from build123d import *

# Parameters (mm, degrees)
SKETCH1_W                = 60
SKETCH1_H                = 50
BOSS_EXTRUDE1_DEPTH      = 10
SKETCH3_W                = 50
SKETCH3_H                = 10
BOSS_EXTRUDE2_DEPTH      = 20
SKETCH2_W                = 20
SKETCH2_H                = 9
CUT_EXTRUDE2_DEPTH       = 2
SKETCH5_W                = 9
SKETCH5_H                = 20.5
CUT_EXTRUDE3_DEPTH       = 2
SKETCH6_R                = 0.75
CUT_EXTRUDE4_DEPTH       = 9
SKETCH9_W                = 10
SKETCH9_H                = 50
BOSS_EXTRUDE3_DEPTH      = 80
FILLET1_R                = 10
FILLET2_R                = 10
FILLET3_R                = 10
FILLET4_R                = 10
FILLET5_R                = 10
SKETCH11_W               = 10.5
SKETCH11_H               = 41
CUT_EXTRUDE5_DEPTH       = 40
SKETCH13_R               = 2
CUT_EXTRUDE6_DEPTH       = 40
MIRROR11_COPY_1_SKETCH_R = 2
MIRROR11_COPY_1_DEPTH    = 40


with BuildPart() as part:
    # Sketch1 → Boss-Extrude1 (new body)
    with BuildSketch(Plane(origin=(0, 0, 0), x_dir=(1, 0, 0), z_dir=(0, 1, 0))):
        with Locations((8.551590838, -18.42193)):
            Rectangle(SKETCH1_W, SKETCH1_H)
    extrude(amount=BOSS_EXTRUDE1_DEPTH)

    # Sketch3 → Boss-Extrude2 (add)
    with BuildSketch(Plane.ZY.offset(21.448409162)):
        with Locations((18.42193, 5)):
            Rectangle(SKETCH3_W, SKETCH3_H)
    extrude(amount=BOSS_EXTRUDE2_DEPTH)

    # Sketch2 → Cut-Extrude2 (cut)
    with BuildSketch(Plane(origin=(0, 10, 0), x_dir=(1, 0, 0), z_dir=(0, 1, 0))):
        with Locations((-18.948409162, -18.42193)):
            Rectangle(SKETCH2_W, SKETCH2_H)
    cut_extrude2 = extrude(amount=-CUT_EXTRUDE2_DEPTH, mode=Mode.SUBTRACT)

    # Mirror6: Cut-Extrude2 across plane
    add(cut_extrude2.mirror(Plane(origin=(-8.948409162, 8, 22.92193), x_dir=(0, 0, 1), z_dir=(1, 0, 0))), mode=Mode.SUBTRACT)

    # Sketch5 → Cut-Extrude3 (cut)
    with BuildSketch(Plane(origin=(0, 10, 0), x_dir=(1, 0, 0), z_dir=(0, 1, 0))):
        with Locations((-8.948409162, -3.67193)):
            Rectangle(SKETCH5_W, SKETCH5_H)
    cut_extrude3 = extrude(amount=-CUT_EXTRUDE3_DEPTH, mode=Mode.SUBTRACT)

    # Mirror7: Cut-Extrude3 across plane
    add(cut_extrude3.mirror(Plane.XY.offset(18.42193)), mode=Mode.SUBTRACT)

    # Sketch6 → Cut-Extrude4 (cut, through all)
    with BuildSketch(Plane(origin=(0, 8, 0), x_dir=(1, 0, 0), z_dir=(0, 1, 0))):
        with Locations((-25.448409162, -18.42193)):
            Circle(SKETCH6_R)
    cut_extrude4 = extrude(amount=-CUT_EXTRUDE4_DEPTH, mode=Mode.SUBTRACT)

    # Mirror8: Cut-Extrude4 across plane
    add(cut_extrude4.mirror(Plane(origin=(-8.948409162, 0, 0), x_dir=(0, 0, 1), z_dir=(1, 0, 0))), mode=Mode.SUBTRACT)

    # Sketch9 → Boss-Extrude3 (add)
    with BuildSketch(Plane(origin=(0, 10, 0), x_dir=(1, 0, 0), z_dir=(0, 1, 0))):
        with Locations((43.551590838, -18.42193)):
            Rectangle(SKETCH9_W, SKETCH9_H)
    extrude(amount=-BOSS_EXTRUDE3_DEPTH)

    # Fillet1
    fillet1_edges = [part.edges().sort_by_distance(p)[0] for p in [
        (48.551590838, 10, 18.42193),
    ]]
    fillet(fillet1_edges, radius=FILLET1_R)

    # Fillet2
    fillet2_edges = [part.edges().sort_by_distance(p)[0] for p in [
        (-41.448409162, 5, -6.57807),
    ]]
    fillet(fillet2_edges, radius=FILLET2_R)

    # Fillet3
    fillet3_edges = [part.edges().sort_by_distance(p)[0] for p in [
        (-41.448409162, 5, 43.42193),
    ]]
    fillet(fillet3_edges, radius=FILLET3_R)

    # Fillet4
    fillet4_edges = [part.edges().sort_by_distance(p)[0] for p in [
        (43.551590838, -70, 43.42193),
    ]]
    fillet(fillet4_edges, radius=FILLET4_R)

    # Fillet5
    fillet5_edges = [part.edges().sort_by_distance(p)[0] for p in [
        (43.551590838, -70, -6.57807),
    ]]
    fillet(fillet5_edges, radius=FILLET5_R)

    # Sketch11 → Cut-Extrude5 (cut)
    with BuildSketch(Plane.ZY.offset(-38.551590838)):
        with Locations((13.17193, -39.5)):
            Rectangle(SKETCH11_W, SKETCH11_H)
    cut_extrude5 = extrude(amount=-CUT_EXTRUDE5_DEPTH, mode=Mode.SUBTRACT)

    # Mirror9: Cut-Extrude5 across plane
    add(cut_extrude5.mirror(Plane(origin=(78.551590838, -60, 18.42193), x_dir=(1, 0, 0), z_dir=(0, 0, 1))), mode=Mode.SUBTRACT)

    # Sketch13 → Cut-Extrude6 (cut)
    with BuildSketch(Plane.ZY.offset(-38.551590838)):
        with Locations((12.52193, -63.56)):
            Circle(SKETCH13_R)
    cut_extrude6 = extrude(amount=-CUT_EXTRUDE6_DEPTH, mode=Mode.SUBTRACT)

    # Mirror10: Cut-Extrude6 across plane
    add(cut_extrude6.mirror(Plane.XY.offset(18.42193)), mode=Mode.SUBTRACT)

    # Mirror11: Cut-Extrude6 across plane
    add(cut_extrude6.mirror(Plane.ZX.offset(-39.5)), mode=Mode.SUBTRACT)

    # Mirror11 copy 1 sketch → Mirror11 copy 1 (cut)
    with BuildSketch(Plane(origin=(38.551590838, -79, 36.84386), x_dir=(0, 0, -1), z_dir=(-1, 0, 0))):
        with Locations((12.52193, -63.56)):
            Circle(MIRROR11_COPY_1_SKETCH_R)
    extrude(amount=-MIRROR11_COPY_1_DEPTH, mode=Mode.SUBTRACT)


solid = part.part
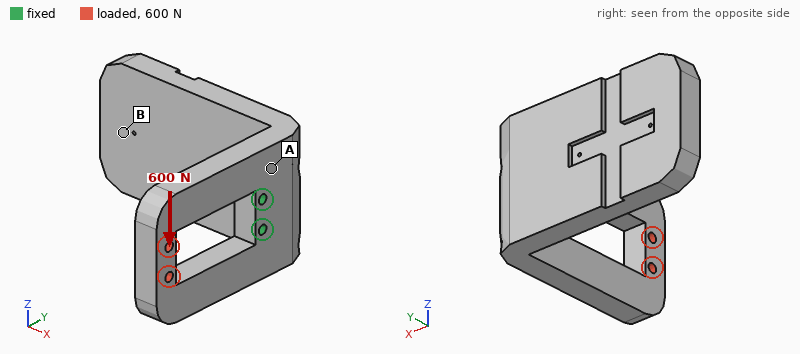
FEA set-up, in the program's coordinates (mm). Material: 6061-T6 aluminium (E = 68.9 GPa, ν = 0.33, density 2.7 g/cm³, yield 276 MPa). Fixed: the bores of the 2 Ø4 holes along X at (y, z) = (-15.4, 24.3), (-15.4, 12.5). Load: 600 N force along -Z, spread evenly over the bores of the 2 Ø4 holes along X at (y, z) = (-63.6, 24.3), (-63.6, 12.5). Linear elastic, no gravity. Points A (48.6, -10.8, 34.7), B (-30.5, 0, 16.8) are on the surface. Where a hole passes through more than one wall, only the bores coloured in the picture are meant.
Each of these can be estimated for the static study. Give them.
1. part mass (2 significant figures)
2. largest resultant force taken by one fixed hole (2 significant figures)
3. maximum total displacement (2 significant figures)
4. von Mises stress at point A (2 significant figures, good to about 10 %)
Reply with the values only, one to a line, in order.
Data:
180 g
1.8 kN
74 µm
9.7 MPa
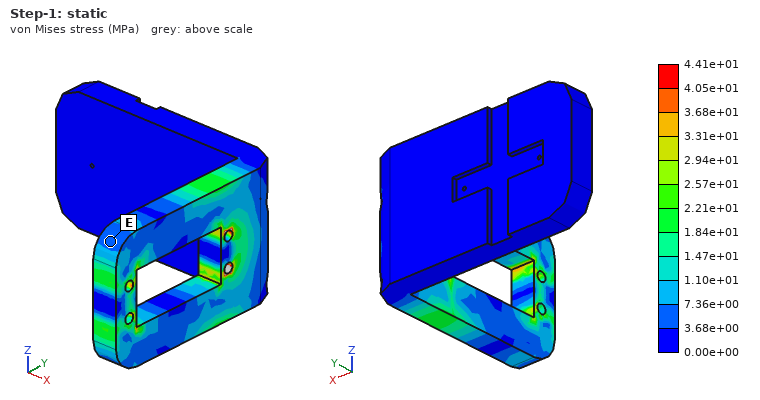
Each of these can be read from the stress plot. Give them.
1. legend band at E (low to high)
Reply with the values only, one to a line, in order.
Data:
3.68e+00 to 7.36e+00 MPa
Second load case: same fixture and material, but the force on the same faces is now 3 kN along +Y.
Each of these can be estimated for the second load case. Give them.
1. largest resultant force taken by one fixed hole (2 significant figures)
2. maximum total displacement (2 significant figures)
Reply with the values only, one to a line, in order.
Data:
1.7 kN
32 µm
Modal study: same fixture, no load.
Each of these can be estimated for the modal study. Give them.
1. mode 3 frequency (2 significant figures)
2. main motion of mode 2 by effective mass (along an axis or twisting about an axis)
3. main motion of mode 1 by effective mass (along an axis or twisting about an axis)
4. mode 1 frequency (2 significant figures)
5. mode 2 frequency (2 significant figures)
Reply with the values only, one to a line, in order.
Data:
1900 Hz
along Z
along Y
800 Hz
1400 Hz
